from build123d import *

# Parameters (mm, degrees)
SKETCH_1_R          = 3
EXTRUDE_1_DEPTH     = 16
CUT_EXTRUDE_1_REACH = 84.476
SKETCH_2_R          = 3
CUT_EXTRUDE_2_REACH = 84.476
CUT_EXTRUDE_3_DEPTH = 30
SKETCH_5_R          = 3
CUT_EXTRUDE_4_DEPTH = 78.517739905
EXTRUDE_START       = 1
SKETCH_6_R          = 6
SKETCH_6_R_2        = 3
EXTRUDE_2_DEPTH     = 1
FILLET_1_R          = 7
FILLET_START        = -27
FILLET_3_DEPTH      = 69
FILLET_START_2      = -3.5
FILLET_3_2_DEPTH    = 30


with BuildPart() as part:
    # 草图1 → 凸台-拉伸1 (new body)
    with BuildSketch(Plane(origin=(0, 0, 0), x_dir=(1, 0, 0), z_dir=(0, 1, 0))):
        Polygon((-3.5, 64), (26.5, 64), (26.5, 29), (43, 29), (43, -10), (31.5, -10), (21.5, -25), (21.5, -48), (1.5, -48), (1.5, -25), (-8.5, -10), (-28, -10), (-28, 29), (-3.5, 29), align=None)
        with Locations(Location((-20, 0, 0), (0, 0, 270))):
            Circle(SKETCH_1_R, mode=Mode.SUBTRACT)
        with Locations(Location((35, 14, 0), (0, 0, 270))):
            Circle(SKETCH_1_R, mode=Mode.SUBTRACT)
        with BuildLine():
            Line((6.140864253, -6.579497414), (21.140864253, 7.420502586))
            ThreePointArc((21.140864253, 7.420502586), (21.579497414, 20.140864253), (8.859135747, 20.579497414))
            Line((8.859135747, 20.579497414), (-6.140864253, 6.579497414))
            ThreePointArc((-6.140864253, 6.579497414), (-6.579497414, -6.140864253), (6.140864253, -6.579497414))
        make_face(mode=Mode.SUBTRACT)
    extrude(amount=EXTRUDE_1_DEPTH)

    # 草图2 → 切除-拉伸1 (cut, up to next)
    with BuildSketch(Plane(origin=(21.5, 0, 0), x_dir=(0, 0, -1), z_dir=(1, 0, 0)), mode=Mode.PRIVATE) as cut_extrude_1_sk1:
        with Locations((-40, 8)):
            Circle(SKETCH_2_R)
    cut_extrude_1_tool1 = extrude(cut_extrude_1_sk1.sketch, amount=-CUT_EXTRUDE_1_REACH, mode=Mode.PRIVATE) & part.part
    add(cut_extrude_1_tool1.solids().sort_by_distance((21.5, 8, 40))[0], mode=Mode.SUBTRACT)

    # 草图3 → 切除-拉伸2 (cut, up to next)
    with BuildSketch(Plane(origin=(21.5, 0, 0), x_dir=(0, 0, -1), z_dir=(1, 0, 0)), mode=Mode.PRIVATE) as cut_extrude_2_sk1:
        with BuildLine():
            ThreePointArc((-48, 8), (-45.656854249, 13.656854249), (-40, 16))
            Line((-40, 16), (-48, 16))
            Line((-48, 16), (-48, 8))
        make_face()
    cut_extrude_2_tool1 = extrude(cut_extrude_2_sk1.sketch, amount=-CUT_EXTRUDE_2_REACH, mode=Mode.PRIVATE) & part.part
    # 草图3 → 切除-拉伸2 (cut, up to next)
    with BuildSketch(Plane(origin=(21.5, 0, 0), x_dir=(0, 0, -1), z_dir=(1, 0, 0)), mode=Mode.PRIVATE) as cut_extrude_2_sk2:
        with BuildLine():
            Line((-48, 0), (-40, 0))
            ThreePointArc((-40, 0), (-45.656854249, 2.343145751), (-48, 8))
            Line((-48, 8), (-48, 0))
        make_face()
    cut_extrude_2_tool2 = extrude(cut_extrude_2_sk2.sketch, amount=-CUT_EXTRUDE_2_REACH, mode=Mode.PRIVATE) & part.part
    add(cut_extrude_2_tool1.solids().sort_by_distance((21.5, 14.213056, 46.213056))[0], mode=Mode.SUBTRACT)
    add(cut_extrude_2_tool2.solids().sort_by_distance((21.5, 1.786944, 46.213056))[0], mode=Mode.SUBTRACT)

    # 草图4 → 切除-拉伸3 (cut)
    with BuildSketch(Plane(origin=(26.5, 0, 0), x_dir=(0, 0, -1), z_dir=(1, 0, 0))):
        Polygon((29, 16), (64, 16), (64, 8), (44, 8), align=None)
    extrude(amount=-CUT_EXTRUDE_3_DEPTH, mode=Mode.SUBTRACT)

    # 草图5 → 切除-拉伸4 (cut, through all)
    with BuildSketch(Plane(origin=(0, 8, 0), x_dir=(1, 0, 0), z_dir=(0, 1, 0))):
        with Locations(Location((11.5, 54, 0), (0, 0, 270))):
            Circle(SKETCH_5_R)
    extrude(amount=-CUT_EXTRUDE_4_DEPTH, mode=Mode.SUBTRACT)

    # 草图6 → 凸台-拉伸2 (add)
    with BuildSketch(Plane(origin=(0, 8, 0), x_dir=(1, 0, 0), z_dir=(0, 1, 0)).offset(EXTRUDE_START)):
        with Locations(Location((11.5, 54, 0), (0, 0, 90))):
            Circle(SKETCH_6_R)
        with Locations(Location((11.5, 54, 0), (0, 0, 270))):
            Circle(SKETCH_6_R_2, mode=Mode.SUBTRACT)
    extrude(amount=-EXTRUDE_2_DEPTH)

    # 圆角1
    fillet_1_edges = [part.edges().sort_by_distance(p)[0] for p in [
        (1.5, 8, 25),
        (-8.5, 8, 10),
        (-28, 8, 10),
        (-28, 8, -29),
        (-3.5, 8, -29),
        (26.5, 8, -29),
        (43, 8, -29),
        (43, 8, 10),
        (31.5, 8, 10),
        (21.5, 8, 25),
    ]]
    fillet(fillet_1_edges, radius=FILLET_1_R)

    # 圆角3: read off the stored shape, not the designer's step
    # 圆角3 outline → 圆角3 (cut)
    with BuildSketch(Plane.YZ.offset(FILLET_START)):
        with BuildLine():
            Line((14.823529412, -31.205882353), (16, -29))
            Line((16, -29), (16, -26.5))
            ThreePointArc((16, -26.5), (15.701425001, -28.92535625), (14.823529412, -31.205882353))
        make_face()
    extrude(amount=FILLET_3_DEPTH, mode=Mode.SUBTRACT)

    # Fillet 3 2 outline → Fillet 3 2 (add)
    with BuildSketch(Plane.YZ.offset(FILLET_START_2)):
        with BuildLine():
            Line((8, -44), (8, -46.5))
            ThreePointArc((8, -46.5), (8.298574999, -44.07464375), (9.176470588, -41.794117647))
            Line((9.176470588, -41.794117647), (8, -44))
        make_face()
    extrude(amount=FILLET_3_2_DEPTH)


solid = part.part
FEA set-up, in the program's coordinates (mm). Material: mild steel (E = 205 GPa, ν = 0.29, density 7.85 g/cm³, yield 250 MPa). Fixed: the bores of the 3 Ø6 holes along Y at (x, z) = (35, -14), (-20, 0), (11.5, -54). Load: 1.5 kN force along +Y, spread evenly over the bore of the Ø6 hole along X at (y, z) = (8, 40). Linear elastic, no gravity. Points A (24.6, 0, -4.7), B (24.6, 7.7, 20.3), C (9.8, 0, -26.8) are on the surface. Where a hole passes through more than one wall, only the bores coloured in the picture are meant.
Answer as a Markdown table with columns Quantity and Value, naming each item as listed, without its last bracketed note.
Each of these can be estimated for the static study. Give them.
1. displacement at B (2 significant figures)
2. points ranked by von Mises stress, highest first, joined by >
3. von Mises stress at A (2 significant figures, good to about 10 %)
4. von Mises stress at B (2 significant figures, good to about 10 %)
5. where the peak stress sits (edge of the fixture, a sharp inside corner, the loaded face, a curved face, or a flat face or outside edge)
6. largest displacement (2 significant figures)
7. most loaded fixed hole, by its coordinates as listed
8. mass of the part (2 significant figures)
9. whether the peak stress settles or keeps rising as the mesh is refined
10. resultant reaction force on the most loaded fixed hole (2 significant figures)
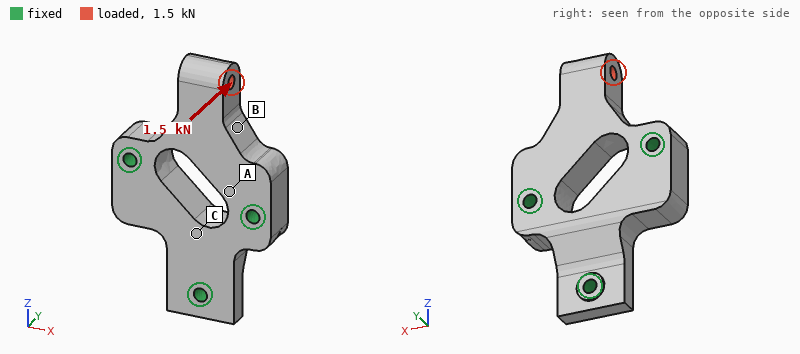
| Quantity | Value |
|---|---|
| displacement at B | 20 µm |
| points ranked by von Mises stress, highest first, joined by > | A > B > C |
| von Mises stress at A | 47 MPa |
| von Mises stress at B | 32 MPa |
| where the peak stress sits | edge of the fixture |
| largest displacement | 56 µm |
| most loaded fixed hole, by its coordinates as listed | (-20, 0) |
| mass of the part | 440 g |
| whether the peak stress settles or keeps rising as the mesh is refined | keeps rising |
| resultant reaction force on the most loaded fixed hole | 1.0 kN |
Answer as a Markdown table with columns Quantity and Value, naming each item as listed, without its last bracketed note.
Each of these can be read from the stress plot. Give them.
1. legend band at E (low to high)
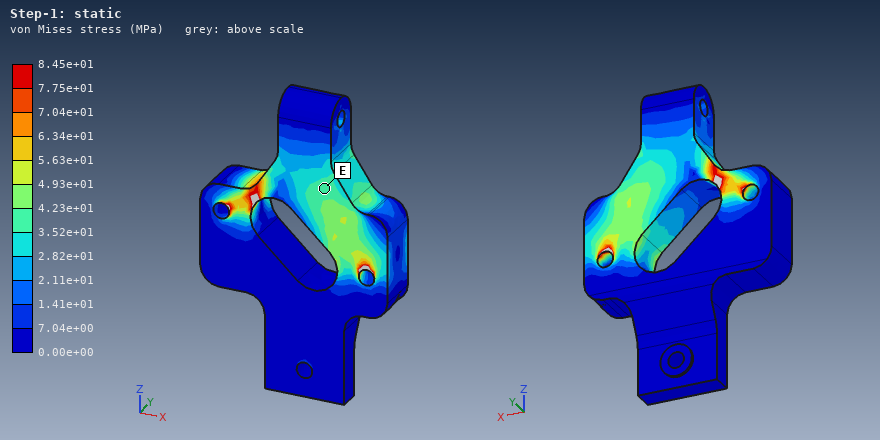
| Quantity | Value |
|---|---|
| legend band at E | 3.52e+01 to 4.23e+01 MPa |
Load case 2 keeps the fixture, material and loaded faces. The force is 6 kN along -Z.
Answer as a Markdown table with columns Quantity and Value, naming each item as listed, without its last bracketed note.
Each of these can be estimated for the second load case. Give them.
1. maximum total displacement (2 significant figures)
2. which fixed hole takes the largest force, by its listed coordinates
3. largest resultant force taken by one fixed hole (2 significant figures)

| Quantity | Value |
|---|---|
| maximum total displacement | 7.3 µm |
| which fixed hole takes the largest force, by its listed coordinates | (35, -14) |
| largest resultant force taken by one fixed hole | 4.2 kN |
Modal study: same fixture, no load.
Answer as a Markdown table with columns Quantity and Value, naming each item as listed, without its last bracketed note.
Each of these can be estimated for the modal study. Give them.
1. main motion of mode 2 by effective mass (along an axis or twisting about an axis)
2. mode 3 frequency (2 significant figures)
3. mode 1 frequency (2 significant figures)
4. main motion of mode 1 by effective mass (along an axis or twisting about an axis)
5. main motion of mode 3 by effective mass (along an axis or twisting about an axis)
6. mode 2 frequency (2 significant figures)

| Quantity | Value |
|---|---|
| main motion of mode 2 by effective mass | along X |
| mode 3 frequency | 14 kHz |
| mode 1 frequency | 4200 Hz |
| main motion of mode 1 by effective mass | along Y |
| main motion of mode 3 by effective mass | along Y |
| mode 2 frequency | 11 kHz |
